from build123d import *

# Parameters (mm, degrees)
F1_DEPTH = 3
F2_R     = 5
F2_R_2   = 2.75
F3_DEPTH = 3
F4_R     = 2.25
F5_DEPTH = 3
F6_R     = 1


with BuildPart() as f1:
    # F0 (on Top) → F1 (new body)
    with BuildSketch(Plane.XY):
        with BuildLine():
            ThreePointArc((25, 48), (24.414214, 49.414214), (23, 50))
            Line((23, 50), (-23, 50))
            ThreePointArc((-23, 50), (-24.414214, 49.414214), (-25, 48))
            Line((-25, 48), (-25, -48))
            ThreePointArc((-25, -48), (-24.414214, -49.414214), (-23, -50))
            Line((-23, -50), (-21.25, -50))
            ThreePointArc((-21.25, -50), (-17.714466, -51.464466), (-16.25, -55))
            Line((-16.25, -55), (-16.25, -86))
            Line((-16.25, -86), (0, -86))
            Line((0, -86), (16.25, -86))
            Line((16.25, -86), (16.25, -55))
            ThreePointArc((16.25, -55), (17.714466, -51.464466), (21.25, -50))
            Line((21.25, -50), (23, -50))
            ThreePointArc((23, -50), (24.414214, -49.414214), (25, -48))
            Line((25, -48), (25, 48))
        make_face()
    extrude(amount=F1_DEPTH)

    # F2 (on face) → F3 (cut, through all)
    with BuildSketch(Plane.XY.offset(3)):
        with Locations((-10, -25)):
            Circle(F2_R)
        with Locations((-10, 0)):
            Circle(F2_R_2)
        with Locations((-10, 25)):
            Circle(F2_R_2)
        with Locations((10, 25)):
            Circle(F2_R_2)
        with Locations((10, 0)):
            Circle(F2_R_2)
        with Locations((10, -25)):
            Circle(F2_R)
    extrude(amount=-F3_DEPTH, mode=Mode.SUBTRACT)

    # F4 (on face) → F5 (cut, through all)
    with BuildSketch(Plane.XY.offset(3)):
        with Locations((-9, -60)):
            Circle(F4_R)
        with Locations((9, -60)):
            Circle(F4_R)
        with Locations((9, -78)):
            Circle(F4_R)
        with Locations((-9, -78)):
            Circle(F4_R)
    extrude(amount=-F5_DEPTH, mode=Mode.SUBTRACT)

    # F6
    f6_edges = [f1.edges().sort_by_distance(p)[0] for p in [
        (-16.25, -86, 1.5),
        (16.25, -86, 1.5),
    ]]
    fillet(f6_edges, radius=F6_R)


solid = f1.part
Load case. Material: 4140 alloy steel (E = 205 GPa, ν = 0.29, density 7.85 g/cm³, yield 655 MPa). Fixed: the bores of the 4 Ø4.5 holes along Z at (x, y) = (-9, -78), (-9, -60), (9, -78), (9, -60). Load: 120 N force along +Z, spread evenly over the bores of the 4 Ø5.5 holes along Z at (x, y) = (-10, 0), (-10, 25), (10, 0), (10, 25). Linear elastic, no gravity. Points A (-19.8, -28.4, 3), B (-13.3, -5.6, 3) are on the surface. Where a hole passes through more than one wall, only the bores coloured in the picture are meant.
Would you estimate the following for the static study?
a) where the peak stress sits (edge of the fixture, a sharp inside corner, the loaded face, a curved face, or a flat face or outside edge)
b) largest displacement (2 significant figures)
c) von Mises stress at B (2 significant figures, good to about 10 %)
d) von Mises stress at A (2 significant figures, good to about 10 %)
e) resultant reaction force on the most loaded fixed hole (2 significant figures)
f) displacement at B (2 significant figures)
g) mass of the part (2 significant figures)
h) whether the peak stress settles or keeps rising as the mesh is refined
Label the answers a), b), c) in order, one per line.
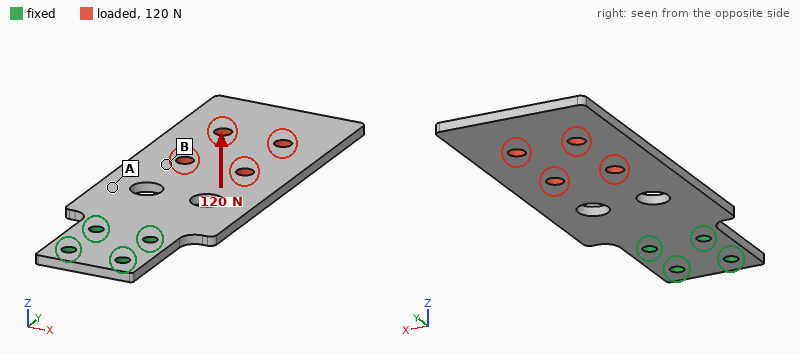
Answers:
a) edge of the fixture
b) 1.4 mm
c) 29 MPa
d) 91 MPa
e) 87 N
f) 0.51 mm
g) 140 g
h) keeps rising
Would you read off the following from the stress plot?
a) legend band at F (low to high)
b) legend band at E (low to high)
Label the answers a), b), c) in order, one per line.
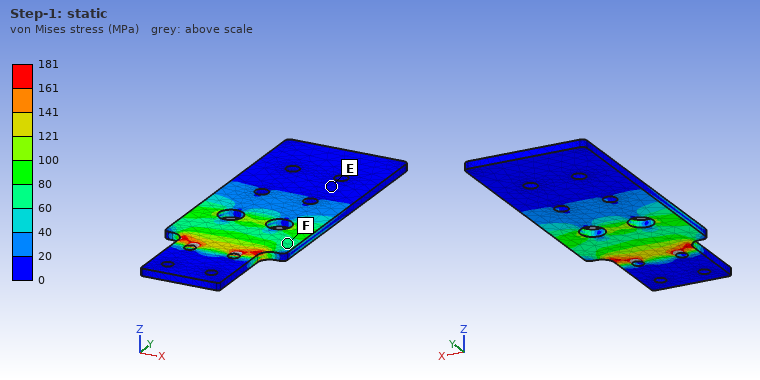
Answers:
a) 60 to 80 MPa
b) 0 to 20 MPa
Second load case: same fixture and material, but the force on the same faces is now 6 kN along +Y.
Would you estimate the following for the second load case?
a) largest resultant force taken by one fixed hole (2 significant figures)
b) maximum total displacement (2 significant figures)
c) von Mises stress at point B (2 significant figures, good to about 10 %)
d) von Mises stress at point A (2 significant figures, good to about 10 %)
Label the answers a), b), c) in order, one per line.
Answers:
a) 2.7 kN
b) 20 µm
c) 43 MPa
d) 48 MPa
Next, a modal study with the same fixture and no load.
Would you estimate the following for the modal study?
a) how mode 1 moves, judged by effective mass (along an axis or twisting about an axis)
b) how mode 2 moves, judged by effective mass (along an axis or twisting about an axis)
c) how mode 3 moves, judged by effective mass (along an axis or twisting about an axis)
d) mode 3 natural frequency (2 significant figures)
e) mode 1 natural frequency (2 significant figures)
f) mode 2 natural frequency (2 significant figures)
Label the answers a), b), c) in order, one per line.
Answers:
a) along Z
b) twisting about Y
c) along Z
d) 1200 Hz
e) 190 Hz
f) 850 Hz
